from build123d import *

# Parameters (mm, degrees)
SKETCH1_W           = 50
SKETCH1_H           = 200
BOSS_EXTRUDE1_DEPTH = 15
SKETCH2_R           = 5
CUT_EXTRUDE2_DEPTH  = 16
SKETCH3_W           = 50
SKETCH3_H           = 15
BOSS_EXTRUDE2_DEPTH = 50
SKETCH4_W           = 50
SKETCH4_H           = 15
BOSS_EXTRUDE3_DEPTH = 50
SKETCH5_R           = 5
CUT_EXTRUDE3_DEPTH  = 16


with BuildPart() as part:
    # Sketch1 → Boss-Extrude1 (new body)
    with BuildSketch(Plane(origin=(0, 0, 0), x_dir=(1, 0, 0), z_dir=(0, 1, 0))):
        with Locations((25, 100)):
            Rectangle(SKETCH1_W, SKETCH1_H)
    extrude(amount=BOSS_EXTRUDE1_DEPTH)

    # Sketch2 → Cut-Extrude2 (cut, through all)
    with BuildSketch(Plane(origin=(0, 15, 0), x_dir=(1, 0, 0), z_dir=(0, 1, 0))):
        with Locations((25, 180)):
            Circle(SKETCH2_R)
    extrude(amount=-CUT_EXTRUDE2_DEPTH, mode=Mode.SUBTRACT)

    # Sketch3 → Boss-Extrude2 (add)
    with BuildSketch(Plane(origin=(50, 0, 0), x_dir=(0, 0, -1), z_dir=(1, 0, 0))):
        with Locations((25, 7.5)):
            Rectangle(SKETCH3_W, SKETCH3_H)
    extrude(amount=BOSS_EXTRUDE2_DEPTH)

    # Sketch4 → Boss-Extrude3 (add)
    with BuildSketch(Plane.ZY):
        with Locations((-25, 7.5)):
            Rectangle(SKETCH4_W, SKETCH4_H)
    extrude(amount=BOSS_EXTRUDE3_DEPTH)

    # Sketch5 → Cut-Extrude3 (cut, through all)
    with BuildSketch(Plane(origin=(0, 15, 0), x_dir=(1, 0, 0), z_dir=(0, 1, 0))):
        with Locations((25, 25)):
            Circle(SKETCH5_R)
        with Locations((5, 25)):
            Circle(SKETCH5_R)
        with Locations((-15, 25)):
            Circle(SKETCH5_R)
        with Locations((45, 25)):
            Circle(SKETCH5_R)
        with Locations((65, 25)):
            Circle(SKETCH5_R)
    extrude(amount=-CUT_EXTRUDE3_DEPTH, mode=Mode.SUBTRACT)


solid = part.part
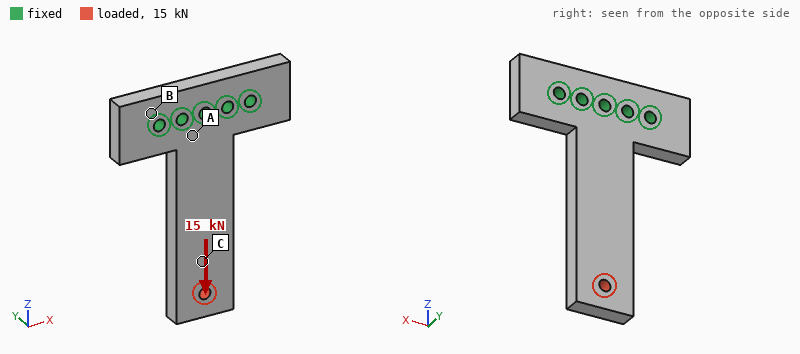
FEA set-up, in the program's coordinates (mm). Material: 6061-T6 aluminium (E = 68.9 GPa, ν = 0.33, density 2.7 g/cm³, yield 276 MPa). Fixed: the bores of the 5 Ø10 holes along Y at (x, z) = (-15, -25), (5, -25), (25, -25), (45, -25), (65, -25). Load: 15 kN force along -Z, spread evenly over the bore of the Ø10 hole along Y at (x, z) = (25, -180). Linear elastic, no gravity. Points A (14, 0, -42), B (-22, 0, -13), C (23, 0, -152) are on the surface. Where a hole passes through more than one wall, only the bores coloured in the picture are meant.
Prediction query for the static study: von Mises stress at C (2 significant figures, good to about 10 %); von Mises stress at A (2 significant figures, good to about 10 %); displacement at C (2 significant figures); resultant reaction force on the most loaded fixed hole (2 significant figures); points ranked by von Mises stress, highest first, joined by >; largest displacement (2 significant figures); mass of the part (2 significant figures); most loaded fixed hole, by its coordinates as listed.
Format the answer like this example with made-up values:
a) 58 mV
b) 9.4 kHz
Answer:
a) 23 MPa
b) 16 MPa
c) 35 µm
d) 4.9 kN
e) C > A > B
f) 51 µm
g) 590 g
h) (25, -25)
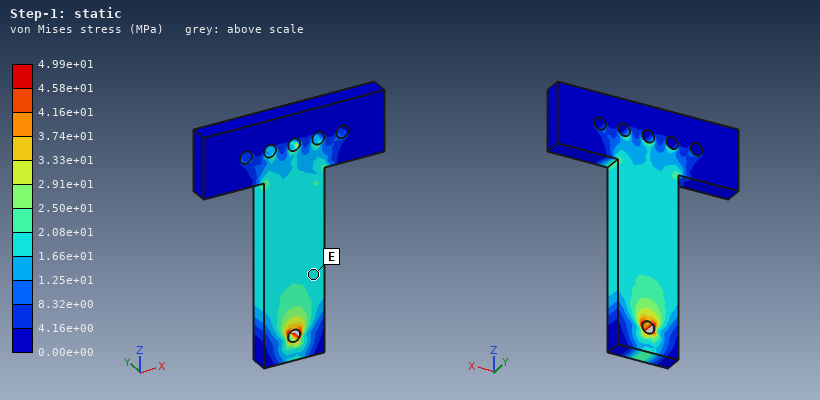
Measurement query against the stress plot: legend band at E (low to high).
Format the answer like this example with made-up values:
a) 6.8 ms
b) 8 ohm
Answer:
a) 1.66e+01 to 2.08e+01 MPa
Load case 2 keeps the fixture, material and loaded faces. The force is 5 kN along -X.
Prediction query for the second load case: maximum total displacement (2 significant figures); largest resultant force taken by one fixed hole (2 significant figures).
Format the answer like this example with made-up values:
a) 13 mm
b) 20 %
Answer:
a) 0.59 mm
b) 9.4 kN
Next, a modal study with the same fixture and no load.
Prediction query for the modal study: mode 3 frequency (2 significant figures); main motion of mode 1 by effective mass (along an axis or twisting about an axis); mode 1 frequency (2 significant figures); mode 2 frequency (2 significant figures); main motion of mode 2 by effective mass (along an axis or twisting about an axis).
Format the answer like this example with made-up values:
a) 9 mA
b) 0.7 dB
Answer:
a) 2600 Hz
b) along Y
c) 450 Hz
d) 1500 Hz
e) along X
